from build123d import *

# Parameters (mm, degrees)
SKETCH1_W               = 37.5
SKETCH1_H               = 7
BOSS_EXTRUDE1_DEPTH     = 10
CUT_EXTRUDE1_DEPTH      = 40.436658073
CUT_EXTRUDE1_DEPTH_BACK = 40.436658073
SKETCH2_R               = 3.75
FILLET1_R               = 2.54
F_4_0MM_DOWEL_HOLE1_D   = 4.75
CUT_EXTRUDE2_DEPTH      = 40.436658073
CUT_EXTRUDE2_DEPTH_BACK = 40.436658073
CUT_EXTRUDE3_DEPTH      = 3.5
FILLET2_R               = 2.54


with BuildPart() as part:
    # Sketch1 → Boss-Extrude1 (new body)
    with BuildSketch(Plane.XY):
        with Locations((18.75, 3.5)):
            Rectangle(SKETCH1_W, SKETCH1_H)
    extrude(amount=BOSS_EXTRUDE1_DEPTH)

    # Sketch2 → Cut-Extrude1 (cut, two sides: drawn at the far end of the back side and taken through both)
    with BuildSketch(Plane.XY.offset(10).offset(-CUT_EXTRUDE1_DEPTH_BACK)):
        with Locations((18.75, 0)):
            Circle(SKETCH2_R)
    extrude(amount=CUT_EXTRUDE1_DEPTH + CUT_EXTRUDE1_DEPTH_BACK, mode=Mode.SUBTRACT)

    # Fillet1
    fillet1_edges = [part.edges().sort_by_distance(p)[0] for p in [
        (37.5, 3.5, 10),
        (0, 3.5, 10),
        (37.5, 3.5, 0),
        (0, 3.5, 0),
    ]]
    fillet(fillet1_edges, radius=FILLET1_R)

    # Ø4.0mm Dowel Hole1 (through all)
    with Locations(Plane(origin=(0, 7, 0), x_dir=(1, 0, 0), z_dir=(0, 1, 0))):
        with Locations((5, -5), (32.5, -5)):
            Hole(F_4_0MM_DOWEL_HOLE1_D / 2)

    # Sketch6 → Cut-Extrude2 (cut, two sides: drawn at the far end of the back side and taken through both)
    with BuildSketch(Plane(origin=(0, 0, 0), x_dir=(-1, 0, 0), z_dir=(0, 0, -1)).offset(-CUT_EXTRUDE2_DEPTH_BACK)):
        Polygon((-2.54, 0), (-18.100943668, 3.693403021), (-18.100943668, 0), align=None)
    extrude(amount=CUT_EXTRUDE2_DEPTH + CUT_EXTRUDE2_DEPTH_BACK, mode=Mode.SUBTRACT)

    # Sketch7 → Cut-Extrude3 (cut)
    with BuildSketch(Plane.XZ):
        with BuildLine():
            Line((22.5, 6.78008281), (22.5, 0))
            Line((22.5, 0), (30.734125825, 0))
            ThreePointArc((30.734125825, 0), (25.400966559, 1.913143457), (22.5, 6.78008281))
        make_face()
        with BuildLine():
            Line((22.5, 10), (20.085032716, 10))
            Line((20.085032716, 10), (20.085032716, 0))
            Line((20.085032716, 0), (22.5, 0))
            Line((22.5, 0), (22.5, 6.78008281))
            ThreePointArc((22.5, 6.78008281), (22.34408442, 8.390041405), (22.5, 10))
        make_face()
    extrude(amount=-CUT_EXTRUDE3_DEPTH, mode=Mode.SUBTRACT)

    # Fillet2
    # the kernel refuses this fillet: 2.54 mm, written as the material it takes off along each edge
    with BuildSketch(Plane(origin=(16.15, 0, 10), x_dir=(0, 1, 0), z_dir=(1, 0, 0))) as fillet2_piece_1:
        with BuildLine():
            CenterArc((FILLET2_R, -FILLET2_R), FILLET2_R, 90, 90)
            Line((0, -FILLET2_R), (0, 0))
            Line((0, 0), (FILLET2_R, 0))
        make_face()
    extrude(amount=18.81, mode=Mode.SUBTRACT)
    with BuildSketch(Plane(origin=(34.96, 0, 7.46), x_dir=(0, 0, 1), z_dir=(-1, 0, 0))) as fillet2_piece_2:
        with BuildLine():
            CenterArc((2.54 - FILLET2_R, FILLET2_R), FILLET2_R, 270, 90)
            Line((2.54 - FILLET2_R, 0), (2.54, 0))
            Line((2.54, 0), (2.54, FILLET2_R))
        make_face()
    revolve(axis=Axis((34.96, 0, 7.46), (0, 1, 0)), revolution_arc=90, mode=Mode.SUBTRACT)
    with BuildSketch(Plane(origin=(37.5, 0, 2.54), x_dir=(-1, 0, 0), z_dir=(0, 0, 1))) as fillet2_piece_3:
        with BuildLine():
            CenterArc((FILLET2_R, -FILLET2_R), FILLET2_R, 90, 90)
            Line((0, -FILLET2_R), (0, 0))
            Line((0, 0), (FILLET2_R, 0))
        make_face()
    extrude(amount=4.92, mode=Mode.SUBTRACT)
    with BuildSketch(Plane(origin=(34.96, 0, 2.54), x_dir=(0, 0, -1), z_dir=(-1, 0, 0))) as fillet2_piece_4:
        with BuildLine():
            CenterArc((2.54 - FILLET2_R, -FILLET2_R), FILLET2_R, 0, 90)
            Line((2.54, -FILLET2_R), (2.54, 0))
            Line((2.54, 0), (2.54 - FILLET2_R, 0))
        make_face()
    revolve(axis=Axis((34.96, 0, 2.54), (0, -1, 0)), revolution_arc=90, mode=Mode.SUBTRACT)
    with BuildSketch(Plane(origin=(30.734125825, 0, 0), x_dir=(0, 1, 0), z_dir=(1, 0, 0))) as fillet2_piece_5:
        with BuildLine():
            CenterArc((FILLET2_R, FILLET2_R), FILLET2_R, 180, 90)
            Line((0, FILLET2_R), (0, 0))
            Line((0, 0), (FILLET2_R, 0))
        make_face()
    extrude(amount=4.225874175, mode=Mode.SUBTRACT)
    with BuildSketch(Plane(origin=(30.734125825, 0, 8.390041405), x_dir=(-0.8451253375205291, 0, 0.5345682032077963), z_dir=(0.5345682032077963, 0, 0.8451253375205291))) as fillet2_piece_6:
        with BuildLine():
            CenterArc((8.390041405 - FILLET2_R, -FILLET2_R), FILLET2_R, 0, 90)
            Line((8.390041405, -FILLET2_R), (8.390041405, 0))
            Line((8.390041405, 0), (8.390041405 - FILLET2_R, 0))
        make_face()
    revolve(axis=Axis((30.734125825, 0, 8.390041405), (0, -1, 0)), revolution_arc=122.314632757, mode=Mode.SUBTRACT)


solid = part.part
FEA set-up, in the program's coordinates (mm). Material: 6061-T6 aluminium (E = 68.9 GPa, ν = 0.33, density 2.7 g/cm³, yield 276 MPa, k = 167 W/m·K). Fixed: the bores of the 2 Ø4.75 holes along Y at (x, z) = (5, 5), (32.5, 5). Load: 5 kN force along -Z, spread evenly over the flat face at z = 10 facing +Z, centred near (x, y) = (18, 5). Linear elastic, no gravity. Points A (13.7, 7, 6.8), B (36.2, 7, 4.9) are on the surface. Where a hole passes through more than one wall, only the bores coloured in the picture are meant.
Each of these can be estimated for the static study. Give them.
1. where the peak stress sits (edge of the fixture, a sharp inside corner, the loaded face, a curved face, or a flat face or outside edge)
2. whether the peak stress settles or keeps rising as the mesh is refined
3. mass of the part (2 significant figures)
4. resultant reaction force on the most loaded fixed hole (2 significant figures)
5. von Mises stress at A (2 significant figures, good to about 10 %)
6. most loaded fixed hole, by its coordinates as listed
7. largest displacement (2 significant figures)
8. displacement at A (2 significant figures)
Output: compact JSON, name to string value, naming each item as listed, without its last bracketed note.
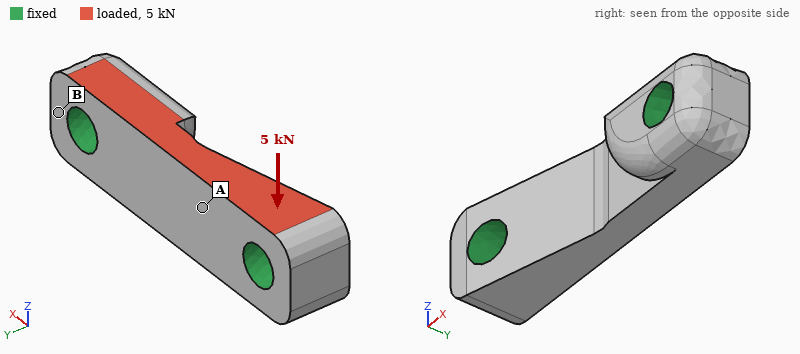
{"where the peak stress sits": "edge of the fixture", "whether the peak stress settles or keeps rising as the mesh is refined": "keeps rising", "mass of the part": "4.9 g", "resultant reaction force on the most loaded fixed hole": "2.7 kN", "von Mises stress at A": "50 MPa", "most loaded fixed hole, by its coordinates as listed": "(5, 5)", "largest displacement": "21 µm", "displacement at A": "15 µm"}
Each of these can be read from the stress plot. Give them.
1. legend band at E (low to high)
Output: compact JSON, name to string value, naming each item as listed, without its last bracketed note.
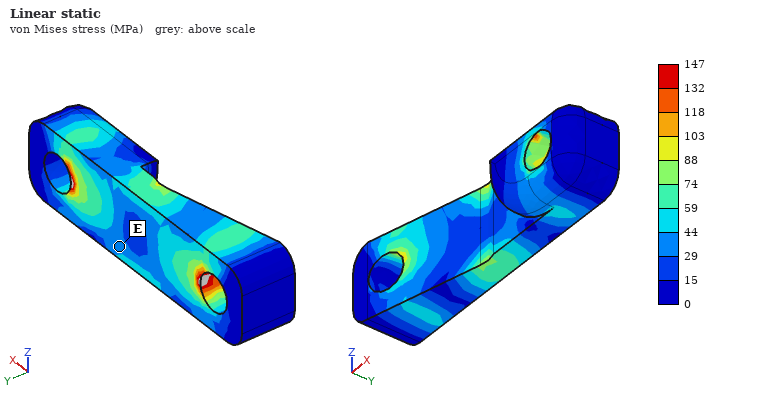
{"legend band at E": "29 to 44 MPa"}
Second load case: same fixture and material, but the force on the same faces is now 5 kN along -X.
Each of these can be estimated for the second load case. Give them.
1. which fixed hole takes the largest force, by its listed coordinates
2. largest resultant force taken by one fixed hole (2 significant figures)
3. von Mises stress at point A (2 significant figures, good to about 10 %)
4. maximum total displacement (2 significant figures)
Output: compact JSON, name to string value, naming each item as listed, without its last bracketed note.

{"which fixed hole takes the largest force, by its listed coordinates": "(5, 5)", "largest resultant force taken by one fixed hole": "2.8 kN", "von Mises stress at point A": "32 MPa", "maximum total displacement": "8.3 µm"}
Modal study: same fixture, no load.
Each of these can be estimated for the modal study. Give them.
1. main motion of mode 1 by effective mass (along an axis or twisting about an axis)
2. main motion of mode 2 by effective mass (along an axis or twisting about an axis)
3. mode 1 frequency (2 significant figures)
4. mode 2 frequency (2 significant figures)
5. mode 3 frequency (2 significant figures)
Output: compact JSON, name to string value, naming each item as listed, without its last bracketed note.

{"main motion of mode 1 by effective mass": "along Y", "main motion of mode 2 by effective mass": "along Z", "mode 1 frequency": "42 kHz", "mode 2 frequency": "47 kHz", "mode 3 frequency": "62 kHz"}
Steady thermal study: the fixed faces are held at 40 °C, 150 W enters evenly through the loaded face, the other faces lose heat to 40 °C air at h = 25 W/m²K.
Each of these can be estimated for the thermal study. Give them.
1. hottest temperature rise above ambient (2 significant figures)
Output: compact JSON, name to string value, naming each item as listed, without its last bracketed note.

{"hottest temperature rise above ambient": "56 K"}
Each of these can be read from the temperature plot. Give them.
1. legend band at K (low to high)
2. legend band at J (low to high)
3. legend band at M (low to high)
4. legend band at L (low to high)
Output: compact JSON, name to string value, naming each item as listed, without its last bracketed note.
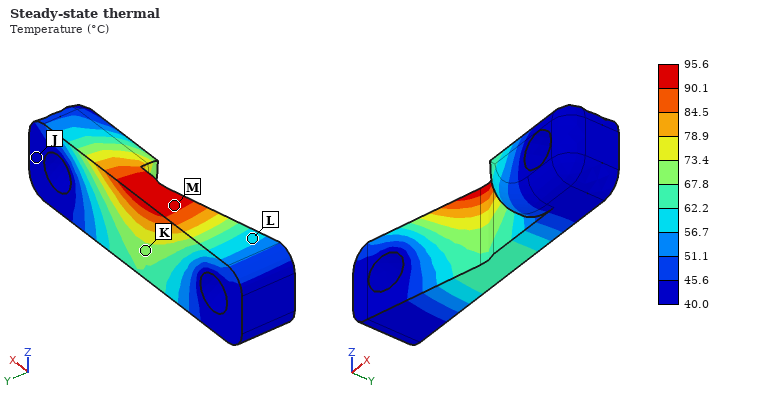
{"legend band at K": "67.8 to 73.4 °C", "legend band at J": "40.0 to 45.6 °C", "legend band at M": "90.1 to 95.6 °C", "legend band at L": "56.7 to 62.2 °C"}
